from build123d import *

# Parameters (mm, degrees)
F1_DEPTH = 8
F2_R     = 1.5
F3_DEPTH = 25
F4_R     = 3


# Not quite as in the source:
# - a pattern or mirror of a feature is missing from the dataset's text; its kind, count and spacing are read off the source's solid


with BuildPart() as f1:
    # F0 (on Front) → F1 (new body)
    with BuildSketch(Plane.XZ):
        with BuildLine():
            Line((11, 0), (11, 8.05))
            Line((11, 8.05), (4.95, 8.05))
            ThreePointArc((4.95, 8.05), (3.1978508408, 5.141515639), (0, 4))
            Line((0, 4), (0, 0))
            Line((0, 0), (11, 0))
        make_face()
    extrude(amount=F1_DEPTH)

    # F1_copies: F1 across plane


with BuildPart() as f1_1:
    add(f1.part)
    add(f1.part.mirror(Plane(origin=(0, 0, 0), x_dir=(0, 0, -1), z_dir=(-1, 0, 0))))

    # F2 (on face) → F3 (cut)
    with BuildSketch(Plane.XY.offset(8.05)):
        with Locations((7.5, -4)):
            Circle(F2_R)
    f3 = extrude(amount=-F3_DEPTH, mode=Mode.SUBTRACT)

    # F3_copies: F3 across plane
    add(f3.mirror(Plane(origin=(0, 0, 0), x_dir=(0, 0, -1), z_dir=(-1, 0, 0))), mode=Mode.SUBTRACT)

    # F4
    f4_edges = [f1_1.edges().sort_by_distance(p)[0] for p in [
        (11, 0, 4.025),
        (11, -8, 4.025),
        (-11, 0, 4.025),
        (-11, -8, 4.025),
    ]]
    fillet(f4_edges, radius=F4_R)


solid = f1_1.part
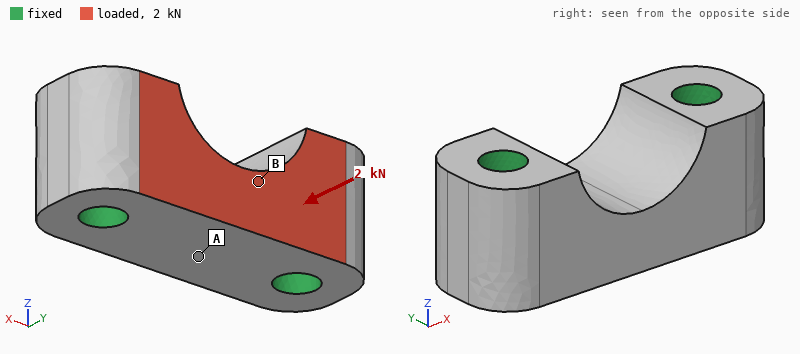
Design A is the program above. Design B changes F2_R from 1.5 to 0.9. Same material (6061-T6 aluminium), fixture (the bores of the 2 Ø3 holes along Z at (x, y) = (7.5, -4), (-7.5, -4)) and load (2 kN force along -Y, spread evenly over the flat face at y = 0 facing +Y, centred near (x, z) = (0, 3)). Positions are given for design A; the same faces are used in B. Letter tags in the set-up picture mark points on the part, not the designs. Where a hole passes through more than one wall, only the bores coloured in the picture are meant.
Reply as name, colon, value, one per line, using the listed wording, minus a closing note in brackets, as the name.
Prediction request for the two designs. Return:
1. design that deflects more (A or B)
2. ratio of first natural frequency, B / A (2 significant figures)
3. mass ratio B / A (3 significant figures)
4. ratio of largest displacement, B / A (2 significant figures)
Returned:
design that deflects more: B
ratio of first natural frequency, B / A: 0.78
mass ratio B / A: 1.07
ratio of largest displacement, B / A: 1.4
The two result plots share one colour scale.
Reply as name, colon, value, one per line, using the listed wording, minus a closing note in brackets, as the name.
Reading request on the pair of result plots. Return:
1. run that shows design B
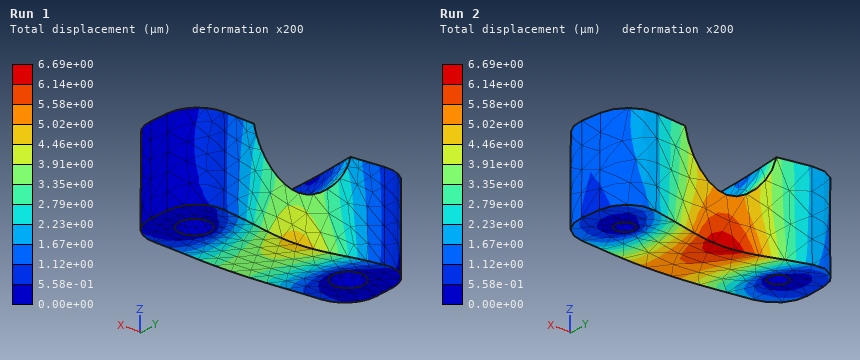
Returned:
run that shows design B: Run 2
